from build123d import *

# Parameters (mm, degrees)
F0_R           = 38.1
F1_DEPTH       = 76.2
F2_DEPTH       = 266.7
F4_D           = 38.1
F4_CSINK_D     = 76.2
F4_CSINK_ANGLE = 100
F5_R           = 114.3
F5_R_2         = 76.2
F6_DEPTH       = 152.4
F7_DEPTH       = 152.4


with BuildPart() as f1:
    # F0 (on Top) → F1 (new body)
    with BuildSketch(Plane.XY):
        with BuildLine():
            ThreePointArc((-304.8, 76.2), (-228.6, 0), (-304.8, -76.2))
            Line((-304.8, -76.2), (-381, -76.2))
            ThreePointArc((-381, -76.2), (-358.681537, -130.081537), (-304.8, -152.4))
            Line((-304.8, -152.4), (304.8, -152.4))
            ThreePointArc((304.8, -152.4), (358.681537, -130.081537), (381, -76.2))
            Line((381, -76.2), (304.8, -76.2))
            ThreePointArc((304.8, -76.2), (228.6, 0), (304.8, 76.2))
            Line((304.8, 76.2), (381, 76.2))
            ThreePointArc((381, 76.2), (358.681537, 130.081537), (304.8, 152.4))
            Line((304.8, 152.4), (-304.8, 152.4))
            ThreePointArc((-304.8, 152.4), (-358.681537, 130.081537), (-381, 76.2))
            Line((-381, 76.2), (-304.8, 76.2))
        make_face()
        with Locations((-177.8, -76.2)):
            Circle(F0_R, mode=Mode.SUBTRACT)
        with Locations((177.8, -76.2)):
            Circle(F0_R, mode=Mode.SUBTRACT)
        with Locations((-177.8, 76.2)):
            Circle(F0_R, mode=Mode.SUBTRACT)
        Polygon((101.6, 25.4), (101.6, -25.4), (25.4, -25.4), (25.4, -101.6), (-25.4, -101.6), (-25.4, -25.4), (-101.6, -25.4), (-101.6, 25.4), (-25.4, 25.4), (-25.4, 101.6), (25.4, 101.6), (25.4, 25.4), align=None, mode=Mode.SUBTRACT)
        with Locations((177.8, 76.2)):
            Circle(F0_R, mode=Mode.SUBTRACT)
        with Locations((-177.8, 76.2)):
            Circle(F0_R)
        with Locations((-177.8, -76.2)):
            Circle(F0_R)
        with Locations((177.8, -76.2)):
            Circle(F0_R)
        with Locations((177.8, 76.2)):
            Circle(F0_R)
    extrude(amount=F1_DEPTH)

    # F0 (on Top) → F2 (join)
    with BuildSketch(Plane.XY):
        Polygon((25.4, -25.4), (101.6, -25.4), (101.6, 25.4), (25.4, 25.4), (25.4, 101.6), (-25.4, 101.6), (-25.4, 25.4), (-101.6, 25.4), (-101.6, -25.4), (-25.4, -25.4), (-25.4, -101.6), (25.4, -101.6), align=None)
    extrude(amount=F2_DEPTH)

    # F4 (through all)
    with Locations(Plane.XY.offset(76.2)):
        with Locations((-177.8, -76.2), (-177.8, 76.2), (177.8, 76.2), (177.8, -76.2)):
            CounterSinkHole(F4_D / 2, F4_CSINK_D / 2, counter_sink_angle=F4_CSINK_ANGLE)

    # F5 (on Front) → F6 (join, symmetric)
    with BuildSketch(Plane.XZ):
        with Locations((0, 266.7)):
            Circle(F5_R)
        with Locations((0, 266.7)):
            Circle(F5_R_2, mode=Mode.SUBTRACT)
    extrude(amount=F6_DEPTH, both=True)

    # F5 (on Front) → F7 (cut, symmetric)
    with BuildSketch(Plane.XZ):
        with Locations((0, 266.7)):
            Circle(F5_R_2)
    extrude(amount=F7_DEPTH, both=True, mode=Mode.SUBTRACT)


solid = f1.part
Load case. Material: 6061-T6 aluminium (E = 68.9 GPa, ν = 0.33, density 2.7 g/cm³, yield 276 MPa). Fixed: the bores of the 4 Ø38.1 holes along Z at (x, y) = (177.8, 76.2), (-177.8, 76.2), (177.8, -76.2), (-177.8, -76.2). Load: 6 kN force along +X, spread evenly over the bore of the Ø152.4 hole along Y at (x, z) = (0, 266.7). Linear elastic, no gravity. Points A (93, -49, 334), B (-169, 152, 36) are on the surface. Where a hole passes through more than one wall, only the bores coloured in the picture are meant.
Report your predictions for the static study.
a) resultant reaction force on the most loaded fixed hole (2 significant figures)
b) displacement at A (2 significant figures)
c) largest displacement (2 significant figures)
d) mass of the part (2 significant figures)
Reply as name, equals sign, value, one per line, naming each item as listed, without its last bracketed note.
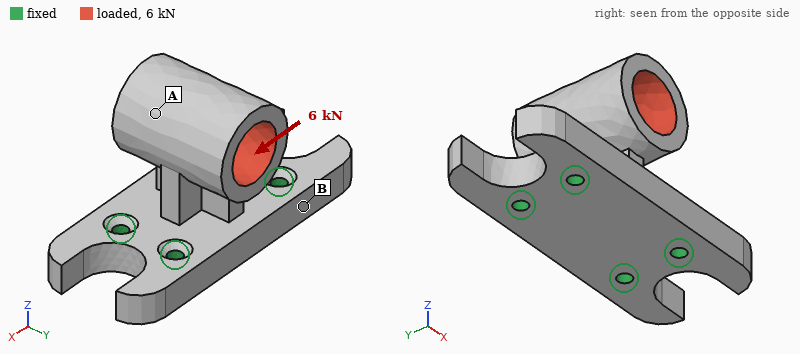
resultant reaction force on the most loaded fixed hole = 2.9 kN
displacement at A = 27 µm
largest displacement = 29 µm
mass of the part = 60 kg
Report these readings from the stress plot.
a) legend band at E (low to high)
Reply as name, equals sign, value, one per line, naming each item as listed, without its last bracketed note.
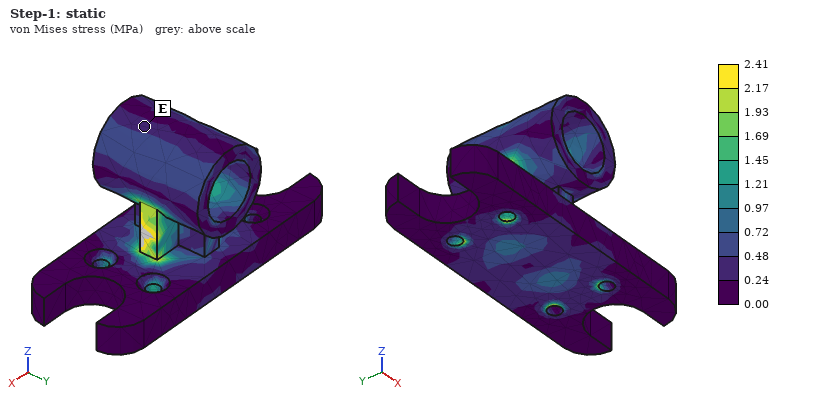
legend band at E = 0.24 to 0.48 MPa
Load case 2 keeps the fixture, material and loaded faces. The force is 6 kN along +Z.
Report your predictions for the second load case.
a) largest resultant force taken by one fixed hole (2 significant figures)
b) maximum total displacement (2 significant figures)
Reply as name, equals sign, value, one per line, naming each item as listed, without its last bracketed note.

largest resultant force taken by one fixed hole = 1.6 kN
maximum total displacement = 4.7 µm
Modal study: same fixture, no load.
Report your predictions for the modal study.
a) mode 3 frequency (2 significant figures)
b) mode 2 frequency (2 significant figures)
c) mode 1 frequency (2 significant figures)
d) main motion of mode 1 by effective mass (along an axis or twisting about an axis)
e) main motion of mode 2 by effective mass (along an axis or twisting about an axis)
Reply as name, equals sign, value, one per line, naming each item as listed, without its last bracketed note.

mode 3 frequency = 900 Hz
mode 2 frequency = 590 Hz
mode 1 frequency = 500 Hz
main motion of mode 1 by effective mass = along Y
main motion of mode 2 by effective mass = along X
